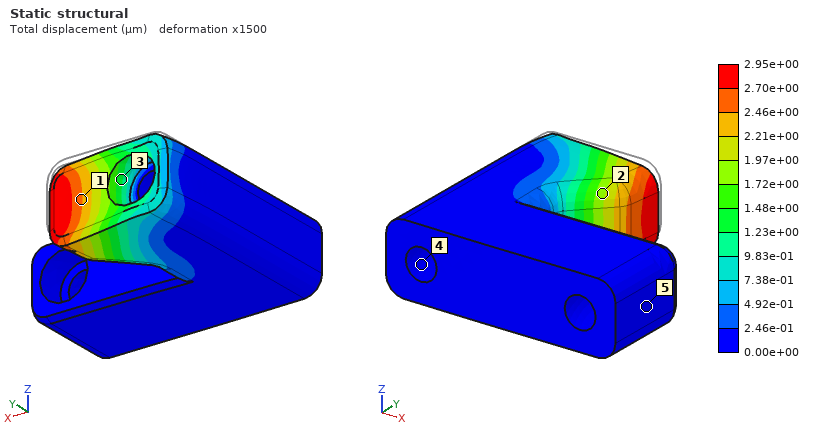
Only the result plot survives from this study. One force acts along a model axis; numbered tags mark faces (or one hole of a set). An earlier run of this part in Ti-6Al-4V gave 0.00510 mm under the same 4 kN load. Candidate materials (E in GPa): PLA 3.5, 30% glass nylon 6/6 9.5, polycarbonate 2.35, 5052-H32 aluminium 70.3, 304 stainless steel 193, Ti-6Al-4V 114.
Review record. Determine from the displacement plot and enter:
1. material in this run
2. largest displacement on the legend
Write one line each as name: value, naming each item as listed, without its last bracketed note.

material in this run: 304 stainless steel
largest displacement on the legend: 2.95e+00 µm
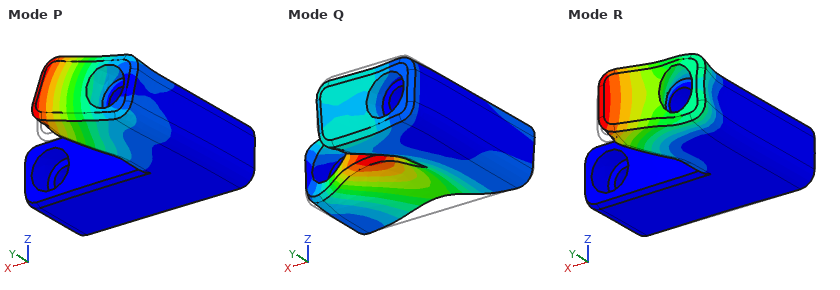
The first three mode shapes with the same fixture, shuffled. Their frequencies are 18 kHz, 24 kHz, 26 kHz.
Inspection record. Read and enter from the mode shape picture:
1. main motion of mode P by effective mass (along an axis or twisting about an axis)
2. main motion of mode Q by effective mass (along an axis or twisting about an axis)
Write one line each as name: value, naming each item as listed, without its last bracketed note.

main motion of mode P by effective mass: along Z
main motion of mode Q by effective mass: along Z
